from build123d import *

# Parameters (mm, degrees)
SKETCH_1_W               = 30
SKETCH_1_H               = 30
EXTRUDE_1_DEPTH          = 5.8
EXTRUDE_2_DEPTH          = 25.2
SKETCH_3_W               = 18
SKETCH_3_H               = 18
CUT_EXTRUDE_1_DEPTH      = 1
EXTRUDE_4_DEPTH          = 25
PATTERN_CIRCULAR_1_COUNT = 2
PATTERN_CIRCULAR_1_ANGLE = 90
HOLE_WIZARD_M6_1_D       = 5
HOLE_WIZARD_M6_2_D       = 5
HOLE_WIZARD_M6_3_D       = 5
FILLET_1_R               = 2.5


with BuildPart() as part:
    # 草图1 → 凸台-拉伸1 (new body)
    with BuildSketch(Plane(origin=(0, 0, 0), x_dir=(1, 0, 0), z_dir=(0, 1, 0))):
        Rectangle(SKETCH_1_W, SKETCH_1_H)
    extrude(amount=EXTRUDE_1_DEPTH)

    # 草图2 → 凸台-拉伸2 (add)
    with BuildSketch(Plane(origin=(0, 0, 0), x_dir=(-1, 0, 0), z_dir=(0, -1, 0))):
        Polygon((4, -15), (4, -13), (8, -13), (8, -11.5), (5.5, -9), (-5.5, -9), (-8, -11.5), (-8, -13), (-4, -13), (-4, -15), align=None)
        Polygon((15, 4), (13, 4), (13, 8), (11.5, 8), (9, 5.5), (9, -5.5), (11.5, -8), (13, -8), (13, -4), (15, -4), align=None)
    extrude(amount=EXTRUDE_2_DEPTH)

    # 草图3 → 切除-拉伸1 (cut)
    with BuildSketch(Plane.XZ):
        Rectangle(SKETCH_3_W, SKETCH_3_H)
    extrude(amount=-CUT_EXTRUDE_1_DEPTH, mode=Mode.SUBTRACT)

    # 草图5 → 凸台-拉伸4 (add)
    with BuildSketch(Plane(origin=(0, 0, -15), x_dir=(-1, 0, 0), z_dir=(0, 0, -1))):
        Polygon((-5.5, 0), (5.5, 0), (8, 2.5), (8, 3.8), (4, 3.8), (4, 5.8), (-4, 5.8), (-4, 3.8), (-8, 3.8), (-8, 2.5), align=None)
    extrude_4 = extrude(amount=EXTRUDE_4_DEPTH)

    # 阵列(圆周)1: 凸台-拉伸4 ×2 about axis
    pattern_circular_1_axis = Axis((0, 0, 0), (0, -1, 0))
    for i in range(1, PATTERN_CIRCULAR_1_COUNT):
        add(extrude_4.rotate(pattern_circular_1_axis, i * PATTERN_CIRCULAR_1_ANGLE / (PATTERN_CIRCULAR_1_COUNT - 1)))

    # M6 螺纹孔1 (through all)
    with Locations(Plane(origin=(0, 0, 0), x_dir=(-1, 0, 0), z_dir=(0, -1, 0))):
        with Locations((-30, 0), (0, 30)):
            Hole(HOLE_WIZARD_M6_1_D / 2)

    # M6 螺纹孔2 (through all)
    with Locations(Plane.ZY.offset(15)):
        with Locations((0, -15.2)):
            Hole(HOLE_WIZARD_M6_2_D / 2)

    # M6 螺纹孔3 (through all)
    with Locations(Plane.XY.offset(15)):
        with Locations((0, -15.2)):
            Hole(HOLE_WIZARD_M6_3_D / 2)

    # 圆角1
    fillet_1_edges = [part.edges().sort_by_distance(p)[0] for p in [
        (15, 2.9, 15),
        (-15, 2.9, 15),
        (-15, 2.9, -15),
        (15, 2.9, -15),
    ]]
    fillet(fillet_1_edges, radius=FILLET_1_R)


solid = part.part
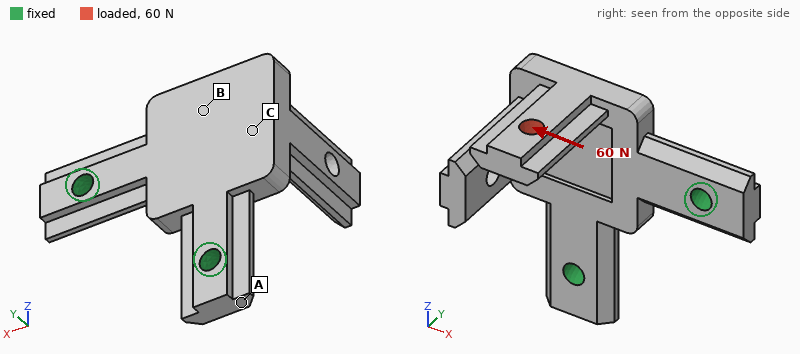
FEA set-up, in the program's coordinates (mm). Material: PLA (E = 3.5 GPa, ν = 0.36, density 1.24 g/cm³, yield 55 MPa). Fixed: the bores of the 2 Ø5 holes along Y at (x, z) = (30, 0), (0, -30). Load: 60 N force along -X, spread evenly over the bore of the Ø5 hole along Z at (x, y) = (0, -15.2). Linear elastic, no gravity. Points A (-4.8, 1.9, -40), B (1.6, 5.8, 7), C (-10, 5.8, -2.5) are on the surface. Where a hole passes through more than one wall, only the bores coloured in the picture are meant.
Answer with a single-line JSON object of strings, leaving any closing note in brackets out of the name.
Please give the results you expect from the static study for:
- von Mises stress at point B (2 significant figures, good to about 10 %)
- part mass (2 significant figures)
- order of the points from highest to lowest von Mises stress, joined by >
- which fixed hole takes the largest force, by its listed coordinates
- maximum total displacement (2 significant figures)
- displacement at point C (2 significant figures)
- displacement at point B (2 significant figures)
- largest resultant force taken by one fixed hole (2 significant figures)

{"von Mises stress at point B": "5.5 MPa", "part mass": "14 g", "order of the points from highest to lowest von Mises stress, joined by >": "B > C > A", "which fixed hole takes the largest force, by its listed coordinates": "(30, 0)", "maximum total displacement": "0.79 mm", "displacement at point C": "0.31 mm", "displacement at point B": "0.23 mm", "largest resultant force taken by one fixed hole": "70 N"}
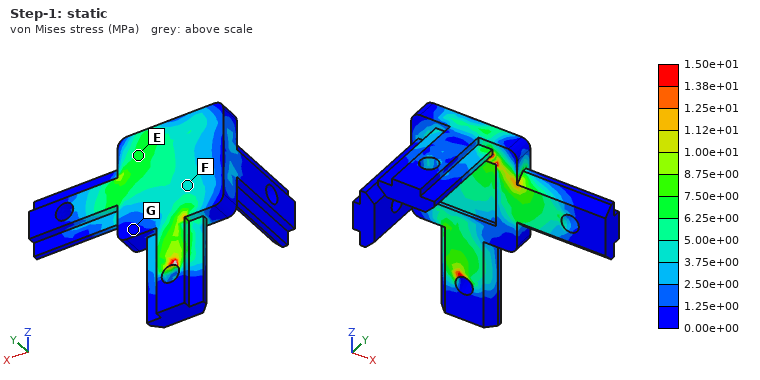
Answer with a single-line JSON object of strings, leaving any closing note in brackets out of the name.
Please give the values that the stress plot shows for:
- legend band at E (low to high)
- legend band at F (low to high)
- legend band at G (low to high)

{"legend band at E": "6.25e+00 to 7.50e+00 MPa", "legend band at F": "3.75e+00 to 5.00e+00 MPa", "legend band at G": "0.00e+00 to 1.25e+00 MPa"}
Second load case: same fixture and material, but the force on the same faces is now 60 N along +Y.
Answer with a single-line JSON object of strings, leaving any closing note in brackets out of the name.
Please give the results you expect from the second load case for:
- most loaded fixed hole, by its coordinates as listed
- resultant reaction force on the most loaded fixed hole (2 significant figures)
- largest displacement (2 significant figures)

{"most loaded fixed hole, by its coordinates as listed": "(30, 0)", "resultant reaction force on the most loaded fixed hole": "45 N", "largest displacement": "1.0 mm"}
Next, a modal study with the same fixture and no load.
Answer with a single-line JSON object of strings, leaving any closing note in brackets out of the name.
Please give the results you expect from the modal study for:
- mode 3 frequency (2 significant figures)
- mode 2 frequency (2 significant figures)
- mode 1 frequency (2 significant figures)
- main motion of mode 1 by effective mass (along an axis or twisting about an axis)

{"mode 3 frequency": "1600 Hz", "mode 2 frequency": "1100 Hz", "mode 1 frequency": "520 Hz", "main motion of mode 1 by effective mass": "along Y"}
